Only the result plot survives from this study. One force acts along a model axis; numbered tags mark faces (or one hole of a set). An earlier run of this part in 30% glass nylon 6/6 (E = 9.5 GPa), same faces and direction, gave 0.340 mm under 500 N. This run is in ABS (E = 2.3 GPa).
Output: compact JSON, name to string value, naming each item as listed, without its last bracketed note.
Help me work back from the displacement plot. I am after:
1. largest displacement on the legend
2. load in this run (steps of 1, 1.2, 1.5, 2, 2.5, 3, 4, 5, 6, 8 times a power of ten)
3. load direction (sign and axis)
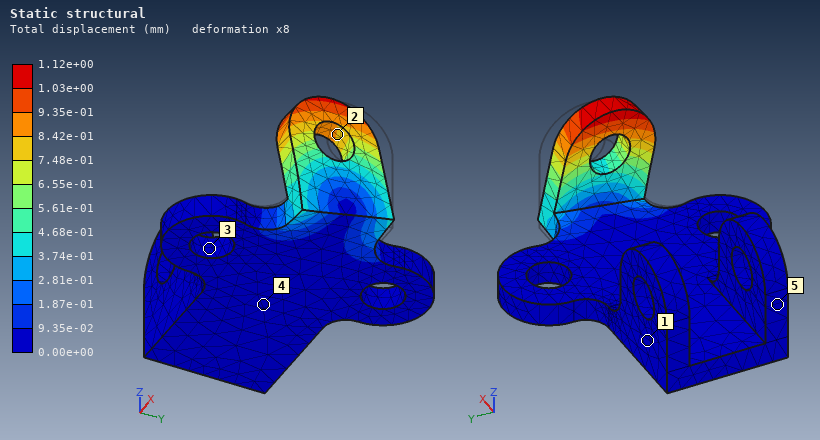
{"largest displacement on the legend": "1.12e+00 mm", "load in this run": "400 N", "load direction": "-Y"}
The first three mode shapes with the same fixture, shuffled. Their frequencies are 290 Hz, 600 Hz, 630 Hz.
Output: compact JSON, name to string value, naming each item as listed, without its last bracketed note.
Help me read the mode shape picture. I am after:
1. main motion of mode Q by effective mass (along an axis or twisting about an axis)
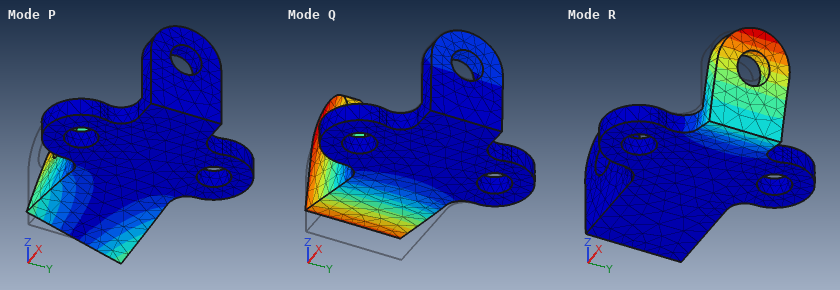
{"main motion of mode Q by effective mass": "along Z"}
